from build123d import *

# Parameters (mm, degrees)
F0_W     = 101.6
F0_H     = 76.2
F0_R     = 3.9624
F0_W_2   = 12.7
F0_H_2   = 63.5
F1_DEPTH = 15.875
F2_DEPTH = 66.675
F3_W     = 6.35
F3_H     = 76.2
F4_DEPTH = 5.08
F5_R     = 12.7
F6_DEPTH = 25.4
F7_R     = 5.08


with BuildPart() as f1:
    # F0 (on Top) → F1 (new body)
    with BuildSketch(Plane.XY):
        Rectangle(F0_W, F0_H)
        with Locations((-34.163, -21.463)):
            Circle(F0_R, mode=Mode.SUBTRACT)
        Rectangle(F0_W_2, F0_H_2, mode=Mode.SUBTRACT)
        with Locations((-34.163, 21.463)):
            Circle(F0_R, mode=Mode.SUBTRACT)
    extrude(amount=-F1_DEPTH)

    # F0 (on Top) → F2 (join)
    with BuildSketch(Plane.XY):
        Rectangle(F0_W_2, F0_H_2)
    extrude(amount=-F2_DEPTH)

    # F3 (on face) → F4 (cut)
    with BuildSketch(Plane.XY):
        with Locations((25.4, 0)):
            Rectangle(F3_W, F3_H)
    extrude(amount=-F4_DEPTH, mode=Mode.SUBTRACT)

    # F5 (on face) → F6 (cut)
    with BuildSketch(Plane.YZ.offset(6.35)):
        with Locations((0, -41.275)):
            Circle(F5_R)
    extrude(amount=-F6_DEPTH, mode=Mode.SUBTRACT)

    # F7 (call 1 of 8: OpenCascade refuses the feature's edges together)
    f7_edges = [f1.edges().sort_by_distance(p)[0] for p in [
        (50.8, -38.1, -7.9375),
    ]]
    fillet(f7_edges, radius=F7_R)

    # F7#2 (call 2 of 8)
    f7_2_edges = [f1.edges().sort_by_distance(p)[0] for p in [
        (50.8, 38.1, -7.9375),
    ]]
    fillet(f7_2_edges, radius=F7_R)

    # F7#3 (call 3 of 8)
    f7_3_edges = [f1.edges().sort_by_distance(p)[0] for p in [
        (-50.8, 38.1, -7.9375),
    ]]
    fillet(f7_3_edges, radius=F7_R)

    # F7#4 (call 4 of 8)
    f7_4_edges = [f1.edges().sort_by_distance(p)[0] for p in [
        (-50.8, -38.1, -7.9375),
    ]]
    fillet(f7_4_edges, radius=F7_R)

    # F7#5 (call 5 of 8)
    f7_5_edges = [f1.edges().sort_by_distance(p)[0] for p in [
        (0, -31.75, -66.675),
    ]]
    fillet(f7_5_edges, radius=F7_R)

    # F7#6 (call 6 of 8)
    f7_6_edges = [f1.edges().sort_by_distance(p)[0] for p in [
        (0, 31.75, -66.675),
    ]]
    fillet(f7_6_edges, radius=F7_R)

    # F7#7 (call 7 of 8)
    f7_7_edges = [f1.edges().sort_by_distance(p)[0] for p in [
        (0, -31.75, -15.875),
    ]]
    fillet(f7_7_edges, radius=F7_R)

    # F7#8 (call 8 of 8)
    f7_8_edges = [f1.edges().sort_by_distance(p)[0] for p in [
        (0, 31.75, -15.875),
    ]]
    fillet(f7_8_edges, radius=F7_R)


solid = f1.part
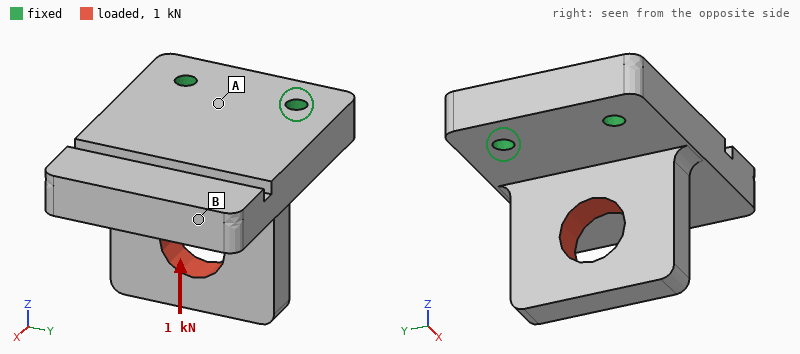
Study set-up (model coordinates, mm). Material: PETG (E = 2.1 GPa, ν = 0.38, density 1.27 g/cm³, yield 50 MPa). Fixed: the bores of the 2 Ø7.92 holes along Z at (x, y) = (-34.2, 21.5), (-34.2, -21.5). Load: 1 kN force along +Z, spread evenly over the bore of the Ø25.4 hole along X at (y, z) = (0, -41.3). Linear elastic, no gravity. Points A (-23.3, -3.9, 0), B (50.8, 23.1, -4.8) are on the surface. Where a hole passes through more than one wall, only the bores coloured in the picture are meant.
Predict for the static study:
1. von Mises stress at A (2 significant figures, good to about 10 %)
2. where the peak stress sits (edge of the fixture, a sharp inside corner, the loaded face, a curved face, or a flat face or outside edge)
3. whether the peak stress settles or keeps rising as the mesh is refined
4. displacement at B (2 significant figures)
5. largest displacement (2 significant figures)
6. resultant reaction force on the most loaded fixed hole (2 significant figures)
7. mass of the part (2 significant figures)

4.7 MPa
edge of the fixture
keeps rising
0.94 mm
0.94 mm
500 N
190 g
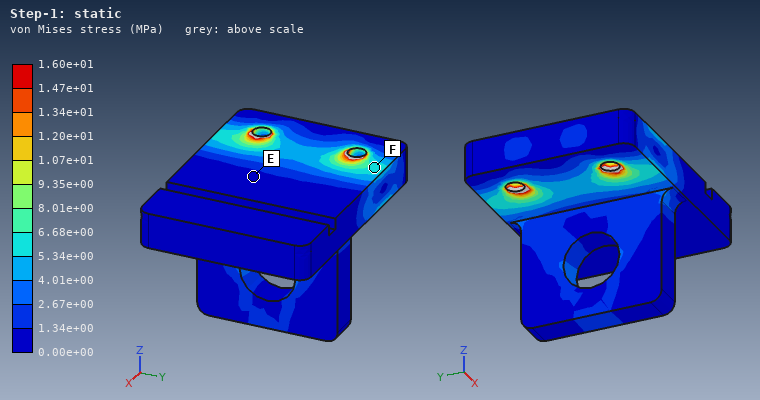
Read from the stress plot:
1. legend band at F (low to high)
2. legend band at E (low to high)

5.34e+00 to 6.68e+00 MPa
0.00e+00 to 1.34e+00 MPa
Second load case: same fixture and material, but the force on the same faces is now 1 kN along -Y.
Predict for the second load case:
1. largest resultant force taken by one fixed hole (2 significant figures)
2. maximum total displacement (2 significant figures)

1.1 kN
0.65 mm
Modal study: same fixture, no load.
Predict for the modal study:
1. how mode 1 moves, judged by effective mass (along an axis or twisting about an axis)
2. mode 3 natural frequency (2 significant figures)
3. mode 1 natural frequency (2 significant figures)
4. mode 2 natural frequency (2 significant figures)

along Z
900 Hz
380 Hz
830 Hz
